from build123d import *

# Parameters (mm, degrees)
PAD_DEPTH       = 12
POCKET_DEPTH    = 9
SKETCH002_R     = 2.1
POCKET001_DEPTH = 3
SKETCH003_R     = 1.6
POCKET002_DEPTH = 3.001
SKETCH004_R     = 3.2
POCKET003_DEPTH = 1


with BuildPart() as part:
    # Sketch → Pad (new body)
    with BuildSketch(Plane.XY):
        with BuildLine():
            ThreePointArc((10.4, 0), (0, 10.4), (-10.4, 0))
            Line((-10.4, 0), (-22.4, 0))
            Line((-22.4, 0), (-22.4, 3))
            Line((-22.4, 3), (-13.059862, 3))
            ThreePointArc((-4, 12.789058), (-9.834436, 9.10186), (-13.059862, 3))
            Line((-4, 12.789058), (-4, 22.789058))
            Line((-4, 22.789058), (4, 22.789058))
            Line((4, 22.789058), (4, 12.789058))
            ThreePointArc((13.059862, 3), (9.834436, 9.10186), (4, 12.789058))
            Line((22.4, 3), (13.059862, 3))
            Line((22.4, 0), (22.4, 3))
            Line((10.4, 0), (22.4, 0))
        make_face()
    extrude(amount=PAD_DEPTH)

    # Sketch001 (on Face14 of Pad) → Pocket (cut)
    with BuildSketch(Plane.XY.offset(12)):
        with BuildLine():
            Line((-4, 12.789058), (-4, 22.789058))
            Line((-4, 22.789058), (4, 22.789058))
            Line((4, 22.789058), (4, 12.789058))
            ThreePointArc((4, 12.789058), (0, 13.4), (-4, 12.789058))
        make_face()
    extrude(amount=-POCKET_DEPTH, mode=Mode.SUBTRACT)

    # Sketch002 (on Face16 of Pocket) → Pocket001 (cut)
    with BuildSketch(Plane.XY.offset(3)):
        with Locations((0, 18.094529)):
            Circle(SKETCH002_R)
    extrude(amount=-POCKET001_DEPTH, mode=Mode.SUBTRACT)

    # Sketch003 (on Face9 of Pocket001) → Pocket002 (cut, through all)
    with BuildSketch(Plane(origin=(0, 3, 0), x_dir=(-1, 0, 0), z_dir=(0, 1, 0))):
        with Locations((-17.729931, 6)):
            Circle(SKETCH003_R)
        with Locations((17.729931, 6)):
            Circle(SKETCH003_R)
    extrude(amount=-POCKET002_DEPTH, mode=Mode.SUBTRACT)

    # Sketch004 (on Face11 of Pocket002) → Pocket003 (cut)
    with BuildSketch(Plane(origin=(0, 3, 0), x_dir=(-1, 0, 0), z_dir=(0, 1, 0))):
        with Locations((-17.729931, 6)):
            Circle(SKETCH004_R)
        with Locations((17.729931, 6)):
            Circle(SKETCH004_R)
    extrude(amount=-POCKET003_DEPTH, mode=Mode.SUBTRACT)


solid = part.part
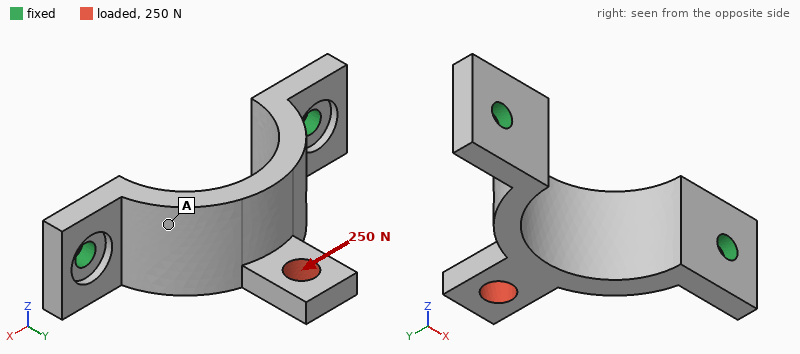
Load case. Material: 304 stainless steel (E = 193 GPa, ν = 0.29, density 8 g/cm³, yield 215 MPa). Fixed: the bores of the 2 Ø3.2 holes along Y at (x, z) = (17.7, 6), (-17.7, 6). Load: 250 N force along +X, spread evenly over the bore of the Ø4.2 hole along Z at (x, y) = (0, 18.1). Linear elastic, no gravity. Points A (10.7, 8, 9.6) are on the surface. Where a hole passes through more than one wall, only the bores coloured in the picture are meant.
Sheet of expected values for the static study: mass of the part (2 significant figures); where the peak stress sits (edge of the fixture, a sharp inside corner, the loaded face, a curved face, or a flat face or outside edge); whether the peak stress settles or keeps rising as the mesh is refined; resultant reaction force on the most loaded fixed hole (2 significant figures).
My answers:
17 g
edge of the fixture
keeps rising
190 N
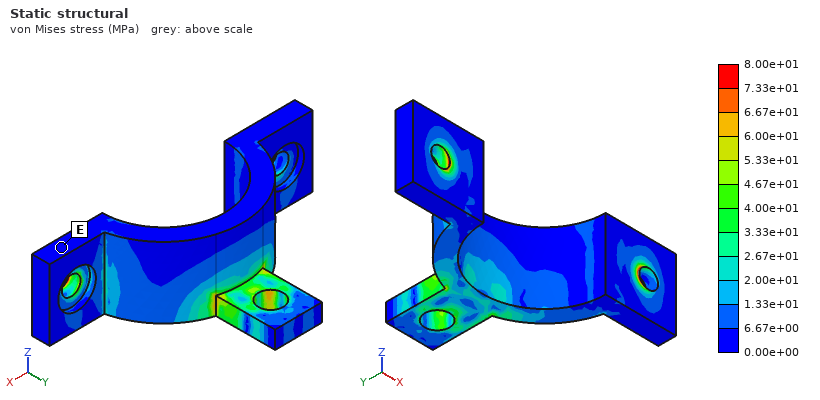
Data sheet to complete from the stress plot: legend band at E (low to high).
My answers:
0.00e+00 to 6.67e+00 MPa
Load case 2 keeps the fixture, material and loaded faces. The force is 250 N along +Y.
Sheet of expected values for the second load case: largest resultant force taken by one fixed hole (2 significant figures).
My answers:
180 N
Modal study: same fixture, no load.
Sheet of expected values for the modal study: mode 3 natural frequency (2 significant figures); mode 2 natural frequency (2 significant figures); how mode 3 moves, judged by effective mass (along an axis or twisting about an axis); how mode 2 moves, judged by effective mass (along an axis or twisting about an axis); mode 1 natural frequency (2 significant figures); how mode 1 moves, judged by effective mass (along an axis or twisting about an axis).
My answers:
19 kHz
16 kHz
along Y
along X
5900 Hz
along Z
